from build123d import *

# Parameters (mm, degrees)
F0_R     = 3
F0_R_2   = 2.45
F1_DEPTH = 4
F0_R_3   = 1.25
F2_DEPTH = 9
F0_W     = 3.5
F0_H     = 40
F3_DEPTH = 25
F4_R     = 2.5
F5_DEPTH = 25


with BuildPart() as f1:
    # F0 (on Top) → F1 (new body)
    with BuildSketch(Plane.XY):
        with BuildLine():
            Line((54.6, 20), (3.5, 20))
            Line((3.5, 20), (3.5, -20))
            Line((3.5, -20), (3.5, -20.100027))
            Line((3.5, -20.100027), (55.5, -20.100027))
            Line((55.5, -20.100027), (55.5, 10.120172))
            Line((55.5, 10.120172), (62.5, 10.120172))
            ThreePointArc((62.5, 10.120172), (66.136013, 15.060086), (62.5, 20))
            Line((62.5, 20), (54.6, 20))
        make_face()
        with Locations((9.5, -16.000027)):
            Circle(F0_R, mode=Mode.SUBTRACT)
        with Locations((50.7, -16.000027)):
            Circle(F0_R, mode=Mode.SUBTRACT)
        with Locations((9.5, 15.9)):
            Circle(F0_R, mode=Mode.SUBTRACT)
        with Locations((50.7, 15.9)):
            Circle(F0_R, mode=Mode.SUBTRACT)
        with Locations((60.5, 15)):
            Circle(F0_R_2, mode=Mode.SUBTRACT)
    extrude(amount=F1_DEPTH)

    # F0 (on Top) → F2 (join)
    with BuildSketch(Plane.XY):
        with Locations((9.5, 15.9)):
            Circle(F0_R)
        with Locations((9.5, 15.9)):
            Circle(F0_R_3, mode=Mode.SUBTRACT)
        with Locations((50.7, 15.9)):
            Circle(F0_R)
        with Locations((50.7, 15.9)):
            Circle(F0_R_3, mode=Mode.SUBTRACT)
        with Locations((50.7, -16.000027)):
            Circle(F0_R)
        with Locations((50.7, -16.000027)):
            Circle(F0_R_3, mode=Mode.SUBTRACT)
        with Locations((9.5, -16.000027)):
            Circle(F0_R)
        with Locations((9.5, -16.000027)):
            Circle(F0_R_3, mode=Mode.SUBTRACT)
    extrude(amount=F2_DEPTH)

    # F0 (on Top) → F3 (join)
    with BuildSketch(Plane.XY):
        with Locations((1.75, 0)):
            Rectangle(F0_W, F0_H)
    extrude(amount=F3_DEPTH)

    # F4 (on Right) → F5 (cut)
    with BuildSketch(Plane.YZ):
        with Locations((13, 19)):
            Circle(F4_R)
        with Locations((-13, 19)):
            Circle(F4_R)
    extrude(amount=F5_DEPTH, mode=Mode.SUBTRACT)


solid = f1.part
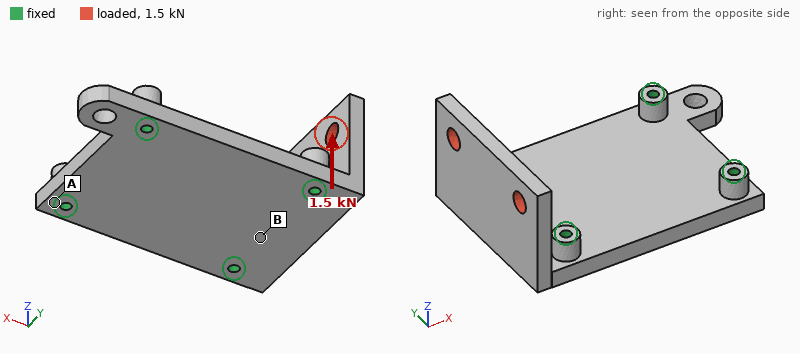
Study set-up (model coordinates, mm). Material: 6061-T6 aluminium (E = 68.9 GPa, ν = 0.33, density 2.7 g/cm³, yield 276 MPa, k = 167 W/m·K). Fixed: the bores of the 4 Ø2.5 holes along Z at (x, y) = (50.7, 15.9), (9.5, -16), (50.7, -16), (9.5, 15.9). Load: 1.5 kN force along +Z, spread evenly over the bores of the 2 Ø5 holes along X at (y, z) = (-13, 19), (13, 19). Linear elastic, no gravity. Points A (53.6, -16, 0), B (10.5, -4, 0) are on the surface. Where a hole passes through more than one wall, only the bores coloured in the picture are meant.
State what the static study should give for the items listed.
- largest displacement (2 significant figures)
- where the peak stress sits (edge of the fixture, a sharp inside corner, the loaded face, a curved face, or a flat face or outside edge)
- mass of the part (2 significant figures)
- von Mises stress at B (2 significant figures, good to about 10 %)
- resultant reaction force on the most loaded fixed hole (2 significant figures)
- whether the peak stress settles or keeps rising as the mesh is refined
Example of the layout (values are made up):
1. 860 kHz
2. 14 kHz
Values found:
1. 89 µm
2. edge of the fixture
3. 33 g
4. 25 MPa
5. 780 N
6. keeps rising
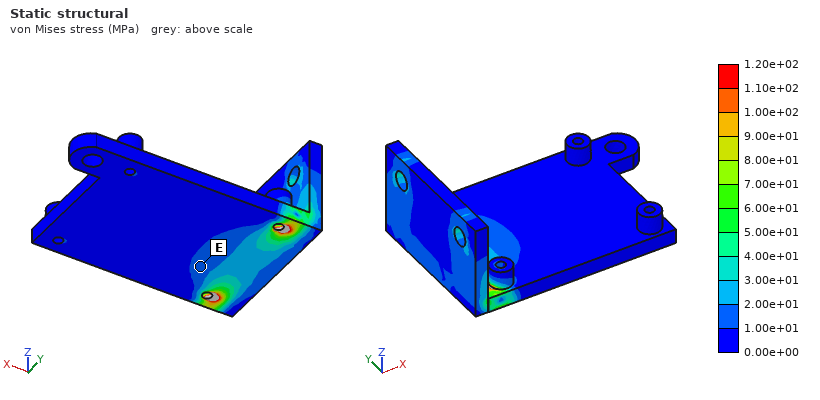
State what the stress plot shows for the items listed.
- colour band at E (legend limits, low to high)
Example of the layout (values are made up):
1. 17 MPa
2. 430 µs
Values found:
1. 1.00e+01 to 2.00e+01 MPa
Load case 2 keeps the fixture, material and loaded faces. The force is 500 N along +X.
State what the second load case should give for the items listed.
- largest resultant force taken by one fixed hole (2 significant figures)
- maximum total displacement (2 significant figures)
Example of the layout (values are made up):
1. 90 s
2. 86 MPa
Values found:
1. 230 N
2. 0.21 mm
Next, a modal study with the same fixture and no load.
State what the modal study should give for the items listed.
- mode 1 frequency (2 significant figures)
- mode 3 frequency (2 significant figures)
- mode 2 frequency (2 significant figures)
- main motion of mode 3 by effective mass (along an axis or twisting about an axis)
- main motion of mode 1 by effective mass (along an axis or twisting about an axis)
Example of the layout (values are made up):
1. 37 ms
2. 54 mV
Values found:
1. 4200 Hz
2. 10 kHz
3. 7800 Hz
4. along Z
5. along X
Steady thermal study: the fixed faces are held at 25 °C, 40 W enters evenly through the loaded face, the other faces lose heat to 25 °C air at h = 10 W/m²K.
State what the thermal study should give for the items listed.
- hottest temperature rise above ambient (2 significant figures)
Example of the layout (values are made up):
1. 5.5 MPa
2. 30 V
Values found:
1. 51 K
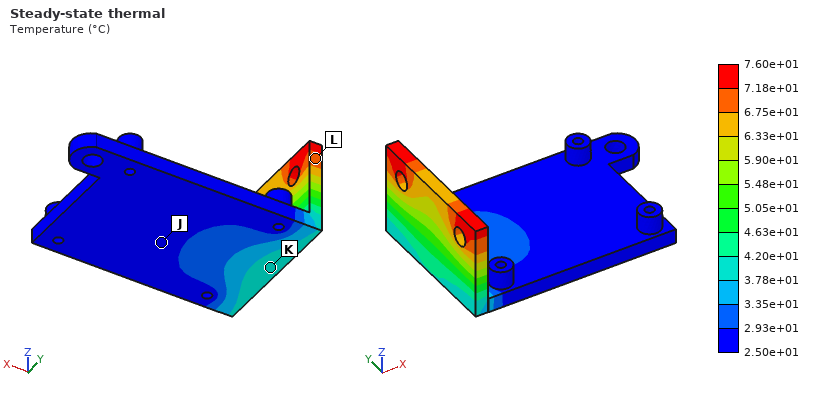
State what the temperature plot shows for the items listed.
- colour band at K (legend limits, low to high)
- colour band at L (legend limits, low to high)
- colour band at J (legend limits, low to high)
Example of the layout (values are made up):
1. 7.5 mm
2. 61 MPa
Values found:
1. 3.78e+01 to 4.20e+01 °C
2. 6.75e+01 to 7.18e+01 °C
3. 2.50e+01 to 2.93e+01 °C
